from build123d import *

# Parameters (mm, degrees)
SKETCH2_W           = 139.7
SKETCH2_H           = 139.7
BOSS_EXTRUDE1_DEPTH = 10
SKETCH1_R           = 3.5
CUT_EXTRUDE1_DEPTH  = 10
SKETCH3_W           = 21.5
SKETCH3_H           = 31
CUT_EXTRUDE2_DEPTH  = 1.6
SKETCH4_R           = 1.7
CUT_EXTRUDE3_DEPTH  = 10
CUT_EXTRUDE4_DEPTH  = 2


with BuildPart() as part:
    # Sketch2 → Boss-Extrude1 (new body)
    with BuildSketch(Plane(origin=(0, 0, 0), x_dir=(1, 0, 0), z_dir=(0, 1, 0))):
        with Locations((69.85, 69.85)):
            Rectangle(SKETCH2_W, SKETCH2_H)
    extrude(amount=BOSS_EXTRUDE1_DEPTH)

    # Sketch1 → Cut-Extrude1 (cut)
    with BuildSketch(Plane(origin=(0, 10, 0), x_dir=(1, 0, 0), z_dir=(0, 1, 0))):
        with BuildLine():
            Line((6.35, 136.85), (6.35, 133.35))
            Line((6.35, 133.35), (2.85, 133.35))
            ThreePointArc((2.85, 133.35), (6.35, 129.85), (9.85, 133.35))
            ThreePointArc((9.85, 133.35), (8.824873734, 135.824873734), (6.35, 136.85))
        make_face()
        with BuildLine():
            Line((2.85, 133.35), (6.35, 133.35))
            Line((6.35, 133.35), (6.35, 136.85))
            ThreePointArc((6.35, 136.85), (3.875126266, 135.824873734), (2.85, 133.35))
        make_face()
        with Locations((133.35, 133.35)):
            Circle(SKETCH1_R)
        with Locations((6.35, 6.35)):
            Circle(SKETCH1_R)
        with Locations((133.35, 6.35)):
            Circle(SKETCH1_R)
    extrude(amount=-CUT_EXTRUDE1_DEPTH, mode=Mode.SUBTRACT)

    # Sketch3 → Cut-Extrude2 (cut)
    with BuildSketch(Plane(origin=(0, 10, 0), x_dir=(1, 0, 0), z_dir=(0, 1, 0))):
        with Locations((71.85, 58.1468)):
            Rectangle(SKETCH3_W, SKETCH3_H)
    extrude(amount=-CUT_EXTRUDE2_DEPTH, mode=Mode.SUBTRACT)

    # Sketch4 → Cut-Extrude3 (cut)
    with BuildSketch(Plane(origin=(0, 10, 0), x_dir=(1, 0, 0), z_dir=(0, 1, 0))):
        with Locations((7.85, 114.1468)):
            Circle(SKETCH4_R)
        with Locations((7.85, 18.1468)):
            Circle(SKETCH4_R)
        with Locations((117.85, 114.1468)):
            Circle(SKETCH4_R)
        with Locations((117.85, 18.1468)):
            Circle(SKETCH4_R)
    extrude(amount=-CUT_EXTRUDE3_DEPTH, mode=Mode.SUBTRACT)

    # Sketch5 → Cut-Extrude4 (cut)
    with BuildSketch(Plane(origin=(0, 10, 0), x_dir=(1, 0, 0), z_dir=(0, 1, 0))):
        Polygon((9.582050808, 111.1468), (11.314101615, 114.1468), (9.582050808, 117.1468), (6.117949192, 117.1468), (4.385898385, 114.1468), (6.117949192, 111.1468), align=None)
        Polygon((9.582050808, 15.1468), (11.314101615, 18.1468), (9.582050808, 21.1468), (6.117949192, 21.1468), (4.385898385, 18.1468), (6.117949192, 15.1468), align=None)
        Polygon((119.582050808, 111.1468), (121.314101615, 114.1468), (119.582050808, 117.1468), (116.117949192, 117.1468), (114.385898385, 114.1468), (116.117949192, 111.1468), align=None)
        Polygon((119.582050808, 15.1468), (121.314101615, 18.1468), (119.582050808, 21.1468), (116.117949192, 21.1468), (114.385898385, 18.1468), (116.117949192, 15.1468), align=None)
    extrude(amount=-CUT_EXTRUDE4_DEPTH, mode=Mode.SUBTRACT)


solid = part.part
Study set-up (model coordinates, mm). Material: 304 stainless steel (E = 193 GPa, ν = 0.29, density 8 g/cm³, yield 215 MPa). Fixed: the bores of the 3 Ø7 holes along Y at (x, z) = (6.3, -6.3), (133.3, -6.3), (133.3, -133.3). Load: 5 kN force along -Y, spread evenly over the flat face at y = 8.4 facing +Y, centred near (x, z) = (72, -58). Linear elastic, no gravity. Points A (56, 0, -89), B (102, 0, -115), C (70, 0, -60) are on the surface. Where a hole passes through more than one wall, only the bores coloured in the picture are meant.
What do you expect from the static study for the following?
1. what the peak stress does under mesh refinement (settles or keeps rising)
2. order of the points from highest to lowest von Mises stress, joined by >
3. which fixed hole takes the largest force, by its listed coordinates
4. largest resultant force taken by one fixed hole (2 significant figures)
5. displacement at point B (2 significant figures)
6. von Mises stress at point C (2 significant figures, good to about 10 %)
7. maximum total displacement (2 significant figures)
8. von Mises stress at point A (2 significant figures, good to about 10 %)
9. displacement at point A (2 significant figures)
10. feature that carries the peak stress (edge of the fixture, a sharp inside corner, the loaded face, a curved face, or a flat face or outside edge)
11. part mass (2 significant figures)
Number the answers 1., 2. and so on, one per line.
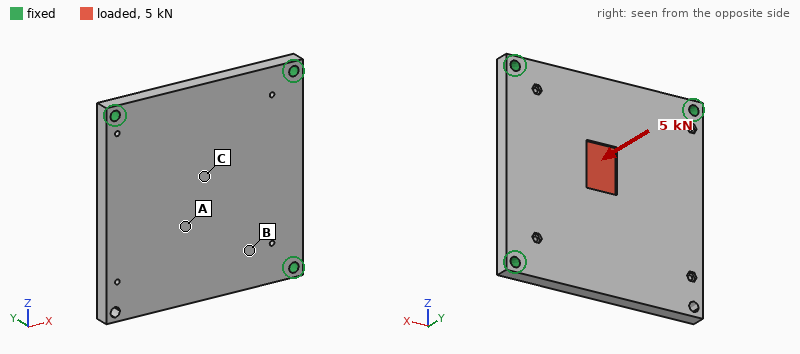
1. keeps rising
2. C > A > B
3. (6.3, -6.3)
4. 2.1 kN
5. 0.053 mm
6. 79 MPa
7. 0.17 mm
8. 42 MPa
9. 0.12 mm
10. edge of the fixture
11. 1.5 kg
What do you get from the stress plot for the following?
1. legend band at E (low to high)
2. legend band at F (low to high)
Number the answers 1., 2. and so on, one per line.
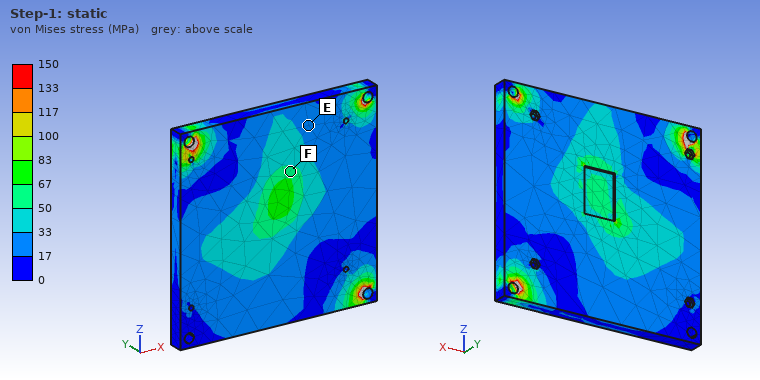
1. 17 to 33 MPa
2. 50 to 67 MPa
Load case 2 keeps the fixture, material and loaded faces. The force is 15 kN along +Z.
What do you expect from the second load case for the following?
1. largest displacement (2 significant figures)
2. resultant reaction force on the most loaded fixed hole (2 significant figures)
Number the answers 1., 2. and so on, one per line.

1. 49 µm
2. 6.4 kN
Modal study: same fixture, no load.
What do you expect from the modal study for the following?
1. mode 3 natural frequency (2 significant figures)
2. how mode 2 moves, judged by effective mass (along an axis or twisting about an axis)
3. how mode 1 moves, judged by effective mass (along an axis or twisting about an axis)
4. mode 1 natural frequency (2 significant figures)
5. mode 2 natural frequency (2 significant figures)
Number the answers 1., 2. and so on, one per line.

1. 2800 Hz
2. along Y
3. along Y
4. 760 Hz
5. 2000 Hz
